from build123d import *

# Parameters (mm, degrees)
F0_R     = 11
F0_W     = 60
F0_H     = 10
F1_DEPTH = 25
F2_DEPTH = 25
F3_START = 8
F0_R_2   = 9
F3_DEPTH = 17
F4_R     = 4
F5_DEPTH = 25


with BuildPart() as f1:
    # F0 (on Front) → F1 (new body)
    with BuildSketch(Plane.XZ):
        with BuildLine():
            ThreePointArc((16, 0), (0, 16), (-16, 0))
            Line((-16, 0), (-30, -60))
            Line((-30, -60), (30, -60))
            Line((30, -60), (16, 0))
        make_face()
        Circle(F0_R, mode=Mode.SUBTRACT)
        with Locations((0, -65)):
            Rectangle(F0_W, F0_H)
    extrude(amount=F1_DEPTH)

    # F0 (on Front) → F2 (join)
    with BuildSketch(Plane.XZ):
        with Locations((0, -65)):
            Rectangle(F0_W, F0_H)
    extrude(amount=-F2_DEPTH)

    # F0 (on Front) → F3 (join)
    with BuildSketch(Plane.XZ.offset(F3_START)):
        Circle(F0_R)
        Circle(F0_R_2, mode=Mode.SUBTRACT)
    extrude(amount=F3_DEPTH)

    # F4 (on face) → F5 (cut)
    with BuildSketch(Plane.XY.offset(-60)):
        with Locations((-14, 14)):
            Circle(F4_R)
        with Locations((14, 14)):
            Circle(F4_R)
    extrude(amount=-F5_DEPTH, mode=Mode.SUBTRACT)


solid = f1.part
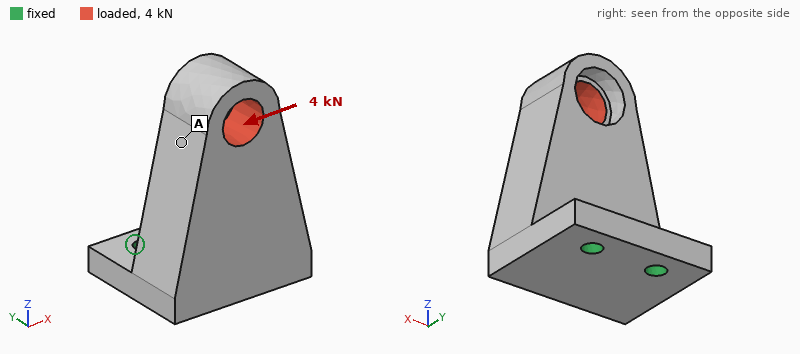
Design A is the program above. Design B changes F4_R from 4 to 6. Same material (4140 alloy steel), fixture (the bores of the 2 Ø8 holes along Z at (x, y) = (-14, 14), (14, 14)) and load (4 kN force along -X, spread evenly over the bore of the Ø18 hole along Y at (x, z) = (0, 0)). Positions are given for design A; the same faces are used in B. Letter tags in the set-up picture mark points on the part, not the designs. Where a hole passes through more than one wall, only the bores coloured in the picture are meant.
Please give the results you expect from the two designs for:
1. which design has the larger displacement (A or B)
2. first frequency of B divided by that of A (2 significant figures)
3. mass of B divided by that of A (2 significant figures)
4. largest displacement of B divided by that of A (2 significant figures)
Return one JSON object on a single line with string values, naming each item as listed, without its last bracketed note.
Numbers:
{"which design has the larger displacement": "A", "first frequency of B divided by that of A": "1.1", "mass of B divided by that of A": "0.99", "largest displacement of B divided by that of A": "0.79"}
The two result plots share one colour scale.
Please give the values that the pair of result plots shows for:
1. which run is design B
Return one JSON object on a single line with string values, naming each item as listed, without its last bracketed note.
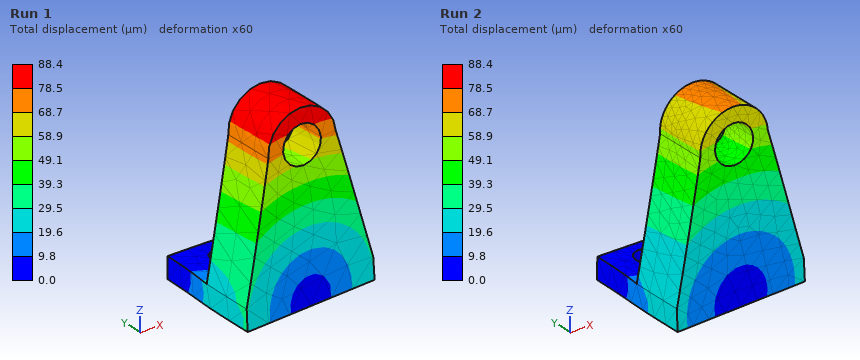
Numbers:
{"which run is design B": "Run 2"}
